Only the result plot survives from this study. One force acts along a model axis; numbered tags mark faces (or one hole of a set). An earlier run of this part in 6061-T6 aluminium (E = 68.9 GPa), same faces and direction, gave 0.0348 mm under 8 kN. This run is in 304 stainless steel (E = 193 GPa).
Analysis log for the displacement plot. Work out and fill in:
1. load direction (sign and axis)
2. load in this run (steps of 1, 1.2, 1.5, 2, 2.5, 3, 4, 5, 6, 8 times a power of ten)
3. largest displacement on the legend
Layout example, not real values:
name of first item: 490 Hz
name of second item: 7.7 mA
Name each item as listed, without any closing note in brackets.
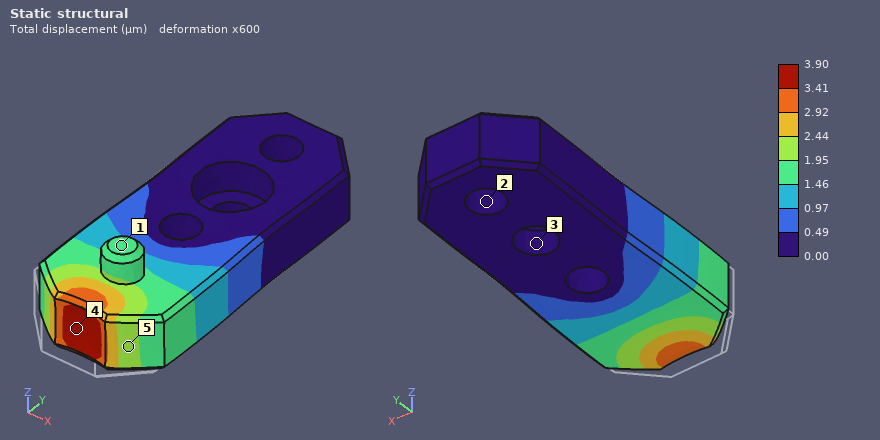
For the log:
load direction: +Y
load in this run: 2.5 kN
largest displacement on the legend: 3.90 µm
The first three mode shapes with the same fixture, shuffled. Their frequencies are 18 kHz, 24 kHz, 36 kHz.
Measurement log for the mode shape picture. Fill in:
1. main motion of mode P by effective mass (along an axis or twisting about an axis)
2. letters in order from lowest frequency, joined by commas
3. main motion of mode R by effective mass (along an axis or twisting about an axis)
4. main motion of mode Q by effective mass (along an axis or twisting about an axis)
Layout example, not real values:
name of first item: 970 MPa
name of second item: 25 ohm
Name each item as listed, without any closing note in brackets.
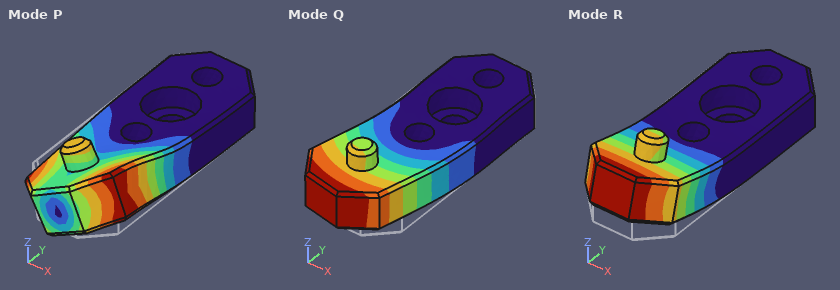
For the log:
main motion of mode P by effective mass: twisting about Y
letters in order from lowest frequency, joined by commas: R, Q, P
main motion of mode R by effective mass: along Z
main motion of mode Q by effective mass: along X
